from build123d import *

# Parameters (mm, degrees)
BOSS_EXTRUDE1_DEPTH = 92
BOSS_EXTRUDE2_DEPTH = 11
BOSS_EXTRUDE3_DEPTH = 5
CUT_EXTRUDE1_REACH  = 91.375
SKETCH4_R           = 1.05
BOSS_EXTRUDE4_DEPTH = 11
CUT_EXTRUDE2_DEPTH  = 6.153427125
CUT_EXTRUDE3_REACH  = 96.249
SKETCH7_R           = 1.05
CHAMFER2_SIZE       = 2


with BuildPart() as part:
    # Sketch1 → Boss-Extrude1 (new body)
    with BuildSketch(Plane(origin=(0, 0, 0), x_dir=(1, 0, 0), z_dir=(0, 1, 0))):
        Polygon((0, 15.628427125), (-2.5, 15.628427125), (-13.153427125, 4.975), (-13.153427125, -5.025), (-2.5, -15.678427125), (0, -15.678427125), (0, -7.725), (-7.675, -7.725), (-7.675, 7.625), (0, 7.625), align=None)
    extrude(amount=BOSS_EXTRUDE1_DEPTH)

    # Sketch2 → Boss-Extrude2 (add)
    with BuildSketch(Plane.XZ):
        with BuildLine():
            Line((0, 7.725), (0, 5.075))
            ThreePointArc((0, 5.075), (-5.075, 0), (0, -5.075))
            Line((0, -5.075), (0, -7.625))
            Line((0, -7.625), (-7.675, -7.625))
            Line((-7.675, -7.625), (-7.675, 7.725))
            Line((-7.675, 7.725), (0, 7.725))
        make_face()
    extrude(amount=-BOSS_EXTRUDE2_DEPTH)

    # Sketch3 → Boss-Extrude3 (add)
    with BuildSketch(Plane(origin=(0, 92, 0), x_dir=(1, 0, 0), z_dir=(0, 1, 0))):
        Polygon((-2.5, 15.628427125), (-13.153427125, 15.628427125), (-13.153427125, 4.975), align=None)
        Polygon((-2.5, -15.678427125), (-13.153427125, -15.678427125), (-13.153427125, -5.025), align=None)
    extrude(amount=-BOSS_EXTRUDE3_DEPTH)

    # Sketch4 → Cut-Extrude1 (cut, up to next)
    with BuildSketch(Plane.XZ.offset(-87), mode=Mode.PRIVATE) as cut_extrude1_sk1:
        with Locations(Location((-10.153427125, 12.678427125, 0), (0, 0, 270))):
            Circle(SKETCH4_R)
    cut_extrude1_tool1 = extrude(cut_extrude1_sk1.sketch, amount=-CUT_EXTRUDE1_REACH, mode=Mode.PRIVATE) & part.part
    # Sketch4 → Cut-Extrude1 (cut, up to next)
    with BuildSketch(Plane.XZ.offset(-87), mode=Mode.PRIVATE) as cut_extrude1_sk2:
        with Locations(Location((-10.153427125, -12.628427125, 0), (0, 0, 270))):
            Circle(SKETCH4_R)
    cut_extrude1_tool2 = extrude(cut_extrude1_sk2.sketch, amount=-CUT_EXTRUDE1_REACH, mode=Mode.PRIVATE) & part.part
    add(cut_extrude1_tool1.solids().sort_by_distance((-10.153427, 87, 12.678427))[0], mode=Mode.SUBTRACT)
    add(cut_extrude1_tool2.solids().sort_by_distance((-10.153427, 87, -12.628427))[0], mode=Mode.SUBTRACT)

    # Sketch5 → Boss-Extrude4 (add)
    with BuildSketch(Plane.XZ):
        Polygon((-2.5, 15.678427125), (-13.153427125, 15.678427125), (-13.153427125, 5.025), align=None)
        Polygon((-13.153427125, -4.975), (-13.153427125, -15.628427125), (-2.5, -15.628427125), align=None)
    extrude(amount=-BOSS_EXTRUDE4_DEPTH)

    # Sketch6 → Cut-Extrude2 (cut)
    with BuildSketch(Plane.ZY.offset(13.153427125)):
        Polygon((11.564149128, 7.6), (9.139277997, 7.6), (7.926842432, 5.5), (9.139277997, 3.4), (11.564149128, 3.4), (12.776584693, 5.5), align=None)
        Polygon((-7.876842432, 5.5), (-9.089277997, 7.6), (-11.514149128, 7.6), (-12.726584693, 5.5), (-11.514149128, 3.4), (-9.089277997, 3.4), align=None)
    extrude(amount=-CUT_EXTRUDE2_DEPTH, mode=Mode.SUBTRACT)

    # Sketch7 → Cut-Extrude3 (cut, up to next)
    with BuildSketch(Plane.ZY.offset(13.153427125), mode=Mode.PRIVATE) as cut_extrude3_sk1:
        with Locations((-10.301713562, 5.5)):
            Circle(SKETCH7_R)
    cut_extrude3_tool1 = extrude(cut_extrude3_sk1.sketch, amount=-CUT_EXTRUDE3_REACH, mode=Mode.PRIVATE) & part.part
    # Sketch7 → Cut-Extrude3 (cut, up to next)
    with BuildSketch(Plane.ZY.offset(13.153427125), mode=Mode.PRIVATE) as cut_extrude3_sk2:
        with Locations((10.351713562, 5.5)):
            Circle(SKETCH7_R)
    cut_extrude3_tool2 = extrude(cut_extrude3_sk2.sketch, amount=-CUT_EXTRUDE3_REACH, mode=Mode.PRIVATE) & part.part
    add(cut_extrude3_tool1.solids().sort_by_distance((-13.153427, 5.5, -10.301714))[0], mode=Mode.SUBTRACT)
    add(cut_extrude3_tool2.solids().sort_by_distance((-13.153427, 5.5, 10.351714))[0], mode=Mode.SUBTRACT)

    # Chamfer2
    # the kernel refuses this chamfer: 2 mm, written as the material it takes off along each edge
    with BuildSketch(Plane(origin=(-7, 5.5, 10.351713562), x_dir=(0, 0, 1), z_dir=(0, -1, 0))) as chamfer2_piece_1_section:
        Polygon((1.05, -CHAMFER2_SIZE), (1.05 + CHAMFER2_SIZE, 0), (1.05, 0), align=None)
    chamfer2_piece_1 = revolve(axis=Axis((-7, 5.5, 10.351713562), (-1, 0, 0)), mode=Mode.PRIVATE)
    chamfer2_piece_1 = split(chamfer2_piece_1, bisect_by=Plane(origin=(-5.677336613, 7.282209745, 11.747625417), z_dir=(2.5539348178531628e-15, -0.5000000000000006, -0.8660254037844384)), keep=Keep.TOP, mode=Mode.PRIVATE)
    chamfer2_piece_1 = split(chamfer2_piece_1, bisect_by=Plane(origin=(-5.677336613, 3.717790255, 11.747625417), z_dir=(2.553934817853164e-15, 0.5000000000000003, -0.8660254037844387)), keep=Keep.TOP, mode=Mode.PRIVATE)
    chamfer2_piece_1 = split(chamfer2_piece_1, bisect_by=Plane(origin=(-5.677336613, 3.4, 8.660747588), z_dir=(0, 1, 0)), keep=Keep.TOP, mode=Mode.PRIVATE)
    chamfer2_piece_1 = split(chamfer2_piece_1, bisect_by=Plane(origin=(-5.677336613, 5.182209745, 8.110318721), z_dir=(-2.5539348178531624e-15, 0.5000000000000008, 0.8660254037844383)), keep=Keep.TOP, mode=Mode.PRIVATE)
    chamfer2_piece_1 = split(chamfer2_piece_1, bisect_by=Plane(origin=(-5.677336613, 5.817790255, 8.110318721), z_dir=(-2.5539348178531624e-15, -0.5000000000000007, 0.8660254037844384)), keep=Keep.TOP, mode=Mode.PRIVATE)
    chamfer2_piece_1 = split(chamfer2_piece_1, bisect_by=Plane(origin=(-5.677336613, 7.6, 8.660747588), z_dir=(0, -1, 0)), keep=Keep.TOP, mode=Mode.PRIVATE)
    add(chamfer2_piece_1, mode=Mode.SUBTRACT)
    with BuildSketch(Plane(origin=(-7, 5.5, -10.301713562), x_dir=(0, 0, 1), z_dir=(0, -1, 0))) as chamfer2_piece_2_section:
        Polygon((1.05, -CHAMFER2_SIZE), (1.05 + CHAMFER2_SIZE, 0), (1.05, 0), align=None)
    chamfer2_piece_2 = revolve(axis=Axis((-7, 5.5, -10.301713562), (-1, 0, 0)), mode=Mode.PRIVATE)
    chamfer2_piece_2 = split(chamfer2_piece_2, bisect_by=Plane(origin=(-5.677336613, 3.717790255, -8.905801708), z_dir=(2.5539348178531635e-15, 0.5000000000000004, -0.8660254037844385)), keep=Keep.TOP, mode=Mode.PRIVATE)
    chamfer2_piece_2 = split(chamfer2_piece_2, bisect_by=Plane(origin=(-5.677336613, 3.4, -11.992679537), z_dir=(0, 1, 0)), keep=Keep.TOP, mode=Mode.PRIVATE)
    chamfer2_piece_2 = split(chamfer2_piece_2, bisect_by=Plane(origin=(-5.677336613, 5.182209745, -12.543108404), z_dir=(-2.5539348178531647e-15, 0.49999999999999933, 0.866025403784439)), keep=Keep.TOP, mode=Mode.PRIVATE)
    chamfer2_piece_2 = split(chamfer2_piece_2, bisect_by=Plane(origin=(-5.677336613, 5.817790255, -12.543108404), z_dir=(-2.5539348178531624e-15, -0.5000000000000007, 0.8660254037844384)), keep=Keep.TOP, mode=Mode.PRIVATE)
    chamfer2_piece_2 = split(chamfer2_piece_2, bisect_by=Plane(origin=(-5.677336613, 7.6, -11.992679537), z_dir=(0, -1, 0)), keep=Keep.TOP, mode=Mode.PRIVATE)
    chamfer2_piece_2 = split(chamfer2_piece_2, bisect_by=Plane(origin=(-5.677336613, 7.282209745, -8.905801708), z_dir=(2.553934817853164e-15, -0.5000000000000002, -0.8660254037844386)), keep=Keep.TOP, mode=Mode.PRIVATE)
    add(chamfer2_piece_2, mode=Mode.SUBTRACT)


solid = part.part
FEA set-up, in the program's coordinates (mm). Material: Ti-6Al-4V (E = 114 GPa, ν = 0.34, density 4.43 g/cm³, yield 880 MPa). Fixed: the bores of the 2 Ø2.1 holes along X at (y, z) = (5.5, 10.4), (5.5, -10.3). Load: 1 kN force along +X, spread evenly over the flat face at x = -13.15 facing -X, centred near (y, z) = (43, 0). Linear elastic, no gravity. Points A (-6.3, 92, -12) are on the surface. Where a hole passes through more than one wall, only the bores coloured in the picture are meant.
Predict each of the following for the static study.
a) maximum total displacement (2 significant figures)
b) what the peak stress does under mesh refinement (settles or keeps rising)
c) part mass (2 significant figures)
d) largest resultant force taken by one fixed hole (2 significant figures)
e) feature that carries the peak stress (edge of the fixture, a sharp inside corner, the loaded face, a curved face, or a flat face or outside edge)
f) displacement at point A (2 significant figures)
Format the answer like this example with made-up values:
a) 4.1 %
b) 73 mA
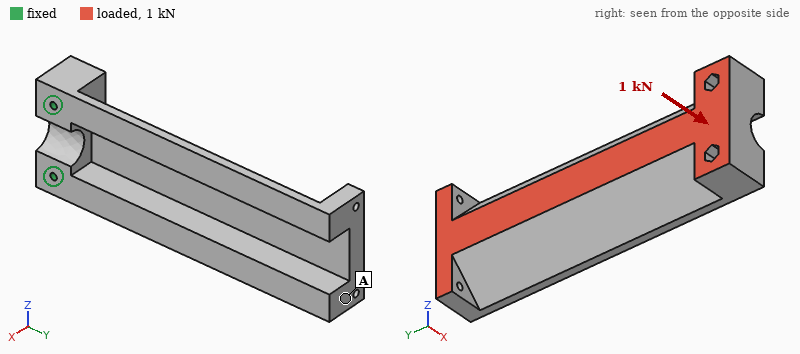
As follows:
a) 0.56 mm
b) keeps rising
c) 84 g
d) 510 N
e) edge of the fixture
f) 0.56 mm
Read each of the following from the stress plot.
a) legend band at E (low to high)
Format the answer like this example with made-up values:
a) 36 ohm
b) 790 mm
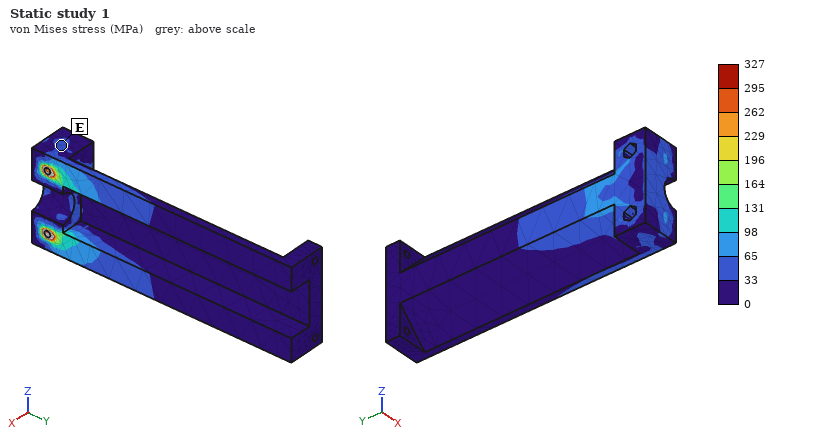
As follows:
a) 33 to 65 MPa
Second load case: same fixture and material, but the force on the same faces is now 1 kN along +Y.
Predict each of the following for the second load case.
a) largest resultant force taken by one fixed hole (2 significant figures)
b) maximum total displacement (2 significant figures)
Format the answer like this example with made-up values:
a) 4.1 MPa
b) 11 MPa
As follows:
a) 500 N
b) 0.13 mm
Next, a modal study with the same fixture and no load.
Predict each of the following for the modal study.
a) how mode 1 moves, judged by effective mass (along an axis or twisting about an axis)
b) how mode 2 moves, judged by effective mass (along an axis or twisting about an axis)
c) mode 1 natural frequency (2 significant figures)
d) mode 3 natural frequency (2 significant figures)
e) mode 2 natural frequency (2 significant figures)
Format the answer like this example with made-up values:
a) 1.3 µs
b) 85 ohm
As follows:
a) along X
b) along Z
c) 900 Hz
d) 3700 Hz
e) 1900 Hz
